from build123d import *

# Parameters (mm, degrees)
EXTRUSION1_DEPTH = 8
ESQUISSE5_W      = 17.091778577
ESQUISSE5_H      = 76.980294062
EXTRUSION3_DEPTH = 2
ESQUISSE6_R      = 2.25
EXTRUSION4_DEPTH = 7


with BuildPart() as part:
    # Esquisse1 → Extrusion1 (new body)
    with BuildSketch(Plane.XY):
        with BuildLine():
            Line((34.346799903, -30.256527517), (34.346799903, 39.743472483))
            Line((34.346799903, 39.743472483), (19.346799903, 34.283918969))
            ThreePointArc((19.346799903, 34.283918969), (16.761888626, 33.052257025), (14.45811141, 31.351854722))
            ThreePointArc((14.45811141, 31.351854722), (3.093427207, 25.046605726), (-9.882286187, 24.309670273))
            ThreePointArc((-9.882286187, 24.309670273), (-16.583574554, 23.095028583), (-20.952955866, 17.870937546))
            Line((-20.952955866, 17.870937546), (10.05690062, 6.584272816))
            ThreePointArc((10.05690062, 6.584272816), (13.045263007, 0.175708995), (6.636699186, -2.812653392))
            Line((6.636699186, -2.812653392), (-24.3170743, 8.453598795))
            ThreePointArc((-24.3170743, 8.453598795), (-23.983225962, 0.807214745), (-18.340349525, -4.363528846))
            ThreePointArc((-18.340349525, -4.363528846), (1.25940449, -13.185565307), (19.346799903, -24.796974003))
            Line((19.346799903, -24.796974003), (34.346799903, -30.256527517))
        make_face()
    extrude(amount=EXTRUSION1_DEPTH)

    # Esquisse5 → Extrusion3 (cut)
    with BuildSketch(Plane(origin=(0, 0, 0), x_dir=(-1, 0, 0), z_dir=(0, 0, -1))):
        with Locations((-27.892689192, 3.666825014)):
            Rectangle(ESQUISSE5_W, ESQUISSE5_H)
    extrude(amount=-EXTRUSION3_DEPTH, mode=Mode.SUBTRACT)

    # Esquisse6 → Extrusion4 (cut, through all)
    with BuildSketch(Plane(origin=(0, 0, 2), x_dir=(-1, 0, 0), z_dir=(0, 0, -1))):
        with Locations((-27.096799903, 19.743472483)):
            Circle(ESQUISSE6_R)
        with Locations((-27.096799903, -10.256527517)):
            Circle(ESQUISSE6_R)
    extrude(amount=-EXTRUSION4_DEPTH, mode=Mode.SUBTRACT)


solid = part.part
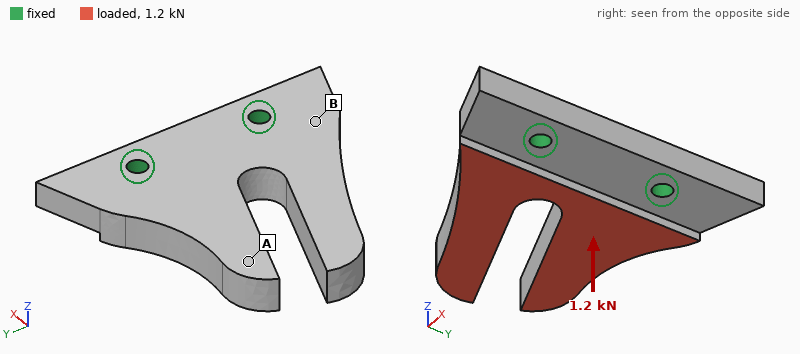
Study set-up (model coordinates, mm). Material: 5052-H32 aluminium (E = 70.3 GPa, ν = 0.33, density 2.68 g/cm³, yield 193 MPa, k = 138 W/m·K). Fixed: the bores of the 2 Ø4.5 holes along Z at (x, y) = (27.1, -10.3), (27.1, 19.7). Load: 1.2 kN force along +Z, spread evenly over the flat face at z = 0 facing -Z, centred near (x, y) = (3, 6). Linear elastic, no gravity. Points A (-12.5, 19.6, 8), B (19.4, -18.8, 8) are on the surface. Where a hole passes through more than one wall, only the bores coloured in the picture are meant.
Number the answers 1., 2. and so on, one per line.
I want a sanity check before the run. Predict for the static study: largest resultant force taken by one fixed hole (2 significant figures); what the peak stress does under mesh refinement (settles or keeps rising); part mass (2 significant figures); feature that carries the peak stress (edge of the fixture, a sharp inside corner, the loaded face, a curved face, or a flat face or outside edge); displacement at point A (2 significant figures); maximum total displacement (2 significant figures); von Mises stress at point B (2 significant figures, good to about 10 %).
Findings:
1. 630 N
2. keeps rising
3. 42 g
4. edge of the fixture
5. 0.16 mm
6. 0.32 mm
7. 51 MPa
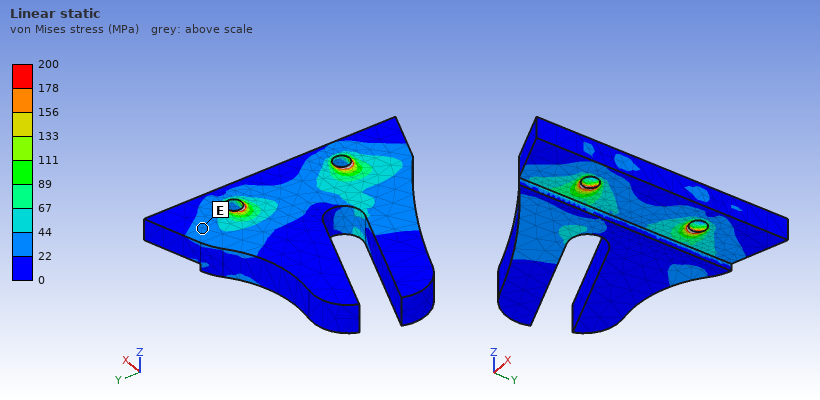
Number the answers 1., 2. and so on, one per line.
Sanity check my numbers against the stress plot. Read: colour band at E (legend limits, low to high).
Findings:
1. 22 to 44 MPa
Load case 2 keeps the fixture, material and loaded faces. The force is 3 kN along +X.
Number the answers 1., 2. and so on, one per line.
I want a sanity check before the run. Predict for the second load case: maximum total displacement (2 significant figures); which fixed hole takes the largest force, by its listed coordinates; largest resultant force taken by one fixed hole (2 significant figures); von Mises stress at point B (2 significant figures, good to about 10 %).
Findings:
1. 0.20 mm
2. (27.1, 19.7)
3. 1.6 kN
4. 33 MPa
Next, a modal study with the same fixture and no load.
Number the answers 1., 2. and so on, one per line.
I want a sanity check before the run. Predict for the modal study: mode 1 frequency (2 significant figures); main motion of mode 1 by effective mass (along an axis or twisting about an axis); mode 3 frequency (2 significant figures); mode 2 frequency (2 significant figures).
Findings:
1. 2600 Hz
2. along Z
3. 5600 Hz
4. 3900 Hz
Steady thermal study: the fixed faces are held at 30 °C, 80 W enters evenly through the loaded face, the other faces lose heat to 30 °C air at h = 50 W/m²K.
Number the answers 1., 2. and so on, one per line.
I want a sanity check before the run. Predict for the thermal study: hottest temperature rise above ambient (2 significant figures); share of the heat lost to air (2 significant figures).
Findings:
1. 62 K
2. 7.9 %
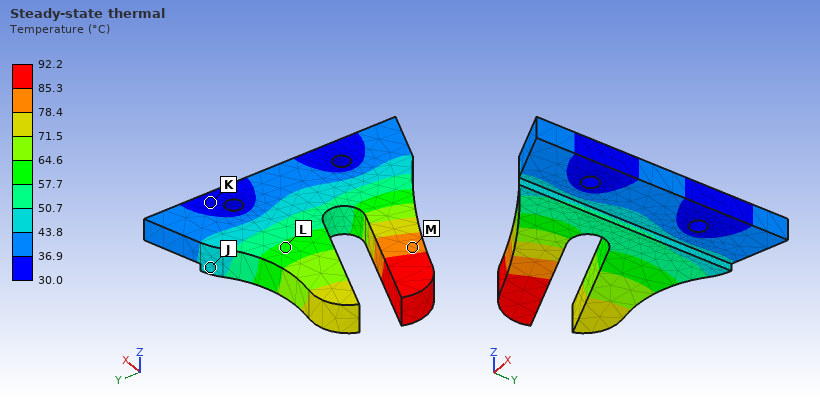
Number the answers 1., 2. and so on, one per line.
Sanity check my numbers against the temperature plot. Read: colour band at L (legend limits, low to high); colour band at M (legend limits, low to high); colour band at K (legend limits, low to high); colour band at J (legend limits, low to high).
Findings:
1. 57.7 to 64.6 °C
2. 78.4 to 85.3 °C
3. 30.0 to 36.9 °C
4. 43.8 to 50.7 °C
